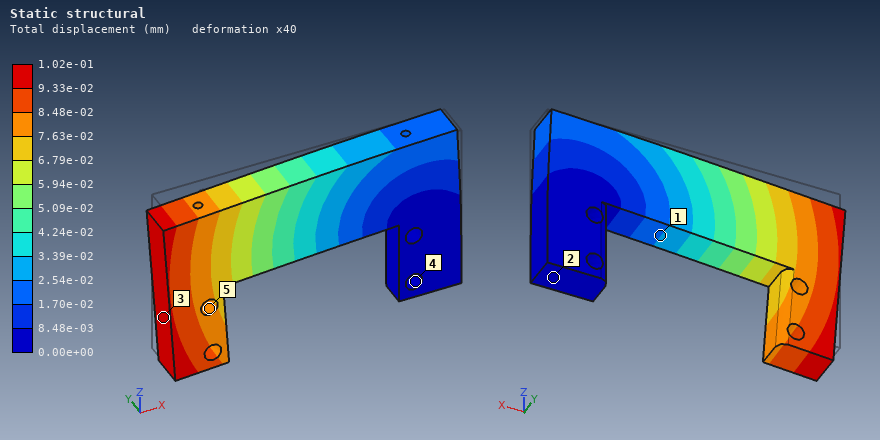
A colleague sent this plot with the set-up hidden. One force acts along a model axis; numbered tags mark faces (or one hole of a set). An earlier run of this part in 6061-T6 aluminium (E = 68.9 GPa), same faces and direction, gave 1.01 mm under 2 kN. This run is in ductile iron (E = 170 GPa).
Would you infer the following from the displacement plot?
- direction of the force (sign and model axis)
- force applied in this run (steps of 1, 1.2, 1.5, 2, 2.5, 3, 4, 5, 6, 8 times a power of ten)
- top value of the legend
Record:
-Z
500 N
1.02e-01 mm
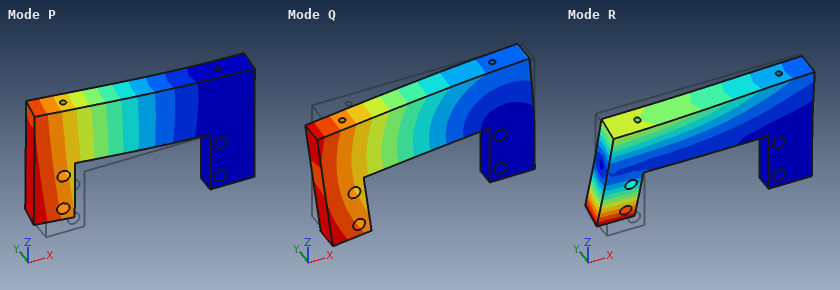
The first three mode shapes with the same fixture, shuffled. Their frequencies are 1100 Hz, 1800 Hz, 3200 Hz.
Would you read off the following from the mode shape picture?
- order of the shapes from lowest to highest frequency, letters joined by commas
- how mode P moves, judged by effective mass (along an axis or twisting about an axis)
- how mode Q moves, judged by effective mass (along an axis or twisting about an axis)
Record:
P, Q, R
along Y
along Z
